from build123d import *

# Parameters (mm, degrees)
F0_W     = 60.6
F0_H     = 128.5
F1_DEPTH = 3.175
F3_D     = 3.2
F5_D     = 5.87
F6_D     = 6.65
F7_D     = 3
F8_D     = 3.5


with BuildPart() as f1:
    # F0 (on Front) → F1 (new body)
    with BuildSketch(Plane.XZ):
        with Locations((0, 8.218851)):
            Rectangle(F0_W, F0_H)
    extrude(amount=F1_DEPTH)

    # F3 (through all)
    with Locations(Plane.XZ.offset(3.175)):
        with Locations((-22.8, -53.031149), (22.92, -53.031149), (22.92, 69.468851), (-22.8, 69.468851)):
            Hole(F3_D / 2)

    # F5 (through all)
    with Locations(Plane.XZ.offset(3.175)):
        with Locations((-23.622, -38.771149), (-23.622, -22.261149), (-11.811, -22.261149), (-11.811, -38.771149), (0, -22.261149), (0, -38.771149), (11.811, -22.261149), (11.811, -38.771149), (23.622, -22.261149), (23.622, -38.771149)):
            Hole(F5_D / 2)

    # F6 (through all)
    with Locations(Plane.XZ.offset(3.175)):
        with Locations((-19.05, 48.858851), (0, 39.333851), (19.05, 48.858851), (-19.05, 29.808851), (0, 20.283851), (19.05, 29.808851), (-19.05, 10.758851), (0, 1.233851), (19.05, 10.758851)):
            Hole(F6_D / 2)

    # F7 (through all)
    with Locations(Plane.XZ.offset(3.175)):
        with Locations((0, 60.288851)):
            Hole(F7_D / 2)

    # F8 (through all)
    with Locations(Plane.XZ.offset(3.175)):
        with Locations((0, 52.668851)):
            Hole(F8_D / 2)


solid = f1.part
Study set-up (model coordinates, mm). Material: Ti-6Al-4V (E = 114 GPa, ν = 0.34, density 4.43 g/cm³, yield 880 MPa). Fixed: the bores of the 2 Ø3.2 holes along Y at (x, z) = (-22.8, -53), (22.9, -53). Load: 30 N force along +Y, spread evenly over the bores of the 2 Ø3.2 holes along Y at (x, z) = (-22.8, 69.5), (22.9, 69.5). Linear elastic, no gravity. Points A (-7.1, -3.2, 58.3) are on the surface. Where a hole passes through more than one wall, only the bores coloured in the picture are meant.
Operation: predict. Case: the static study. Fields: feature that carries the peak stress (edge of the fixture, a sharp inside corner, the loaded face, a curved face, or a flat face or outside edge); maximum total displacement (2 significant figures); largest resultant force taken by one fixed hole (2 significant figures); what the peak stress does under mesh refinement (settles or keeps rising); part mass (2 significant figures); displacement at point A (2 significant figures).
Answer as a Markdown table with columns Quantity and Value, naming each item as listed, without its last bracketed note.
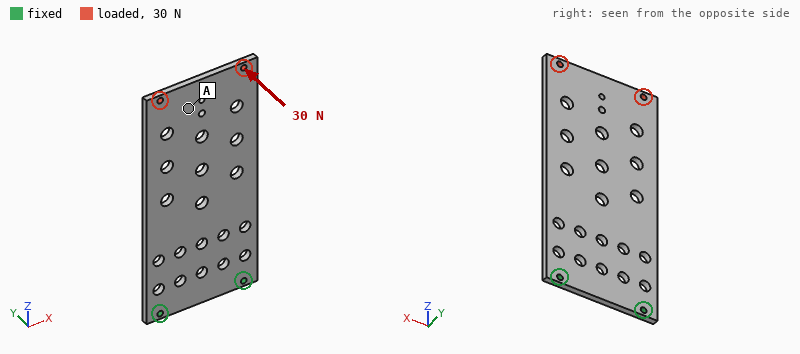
| Quantity | Value |
|---|---|
| feature that carries the peak stress | edge of the fixture |
| maximum total displacement | 1.4 mm |
| largest resultant force taken by one fixed hole | 15 N |
| what the peak stress does under mesh refinement | keeps rising |
| part mass | 100 g |
| displacement at point A | 1.2 mm |
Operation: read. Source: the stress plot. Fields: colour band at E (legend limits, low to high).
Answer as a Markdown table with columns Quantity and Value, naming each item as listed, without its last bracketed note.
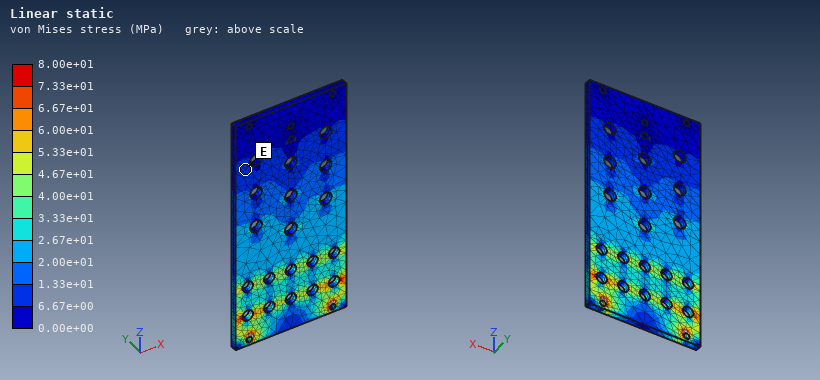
| Quantity | Value |
|---|---|
| colour band at E | 6.67e+00 to 1.33e+01 MPa |
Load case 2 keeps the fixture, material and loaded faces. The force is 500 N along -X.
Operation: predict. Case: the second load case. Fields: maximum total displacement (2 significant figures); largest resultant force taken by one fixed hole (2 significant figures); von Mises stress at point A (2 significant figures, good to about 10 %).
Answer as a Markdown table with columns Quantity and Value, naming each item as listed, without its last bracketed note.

| Quantity | Value |
|---|---|
| maximum total displacement | 85 µm |
| largest resultant force taken by one fixed hole | 1.3 kN |
| von Mises stress at point A | 6.5 MPa |
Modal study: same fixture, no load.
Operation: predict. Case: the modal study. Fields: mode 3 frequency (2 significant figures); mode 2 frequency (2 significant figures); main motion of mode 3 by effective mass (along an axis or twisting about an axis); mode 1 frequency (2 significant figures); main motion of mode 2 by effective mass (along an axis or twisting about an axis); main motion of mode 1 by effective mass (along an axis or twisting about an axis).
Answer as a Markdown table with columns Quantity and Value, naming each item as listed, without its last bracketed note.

| Quantity | Value |
|---|---|
| mode 3 frequency | 940 Hz |
| mode 2 frequency | 690 Hz |
| main motion of mode 3 by effective mass | along Y |
| mode 1 frequency | 140 Hz |
| main motion of mode 2 by effective mass | twisting about Z |
| main motion of mode 1 by effective mass | along Y |
